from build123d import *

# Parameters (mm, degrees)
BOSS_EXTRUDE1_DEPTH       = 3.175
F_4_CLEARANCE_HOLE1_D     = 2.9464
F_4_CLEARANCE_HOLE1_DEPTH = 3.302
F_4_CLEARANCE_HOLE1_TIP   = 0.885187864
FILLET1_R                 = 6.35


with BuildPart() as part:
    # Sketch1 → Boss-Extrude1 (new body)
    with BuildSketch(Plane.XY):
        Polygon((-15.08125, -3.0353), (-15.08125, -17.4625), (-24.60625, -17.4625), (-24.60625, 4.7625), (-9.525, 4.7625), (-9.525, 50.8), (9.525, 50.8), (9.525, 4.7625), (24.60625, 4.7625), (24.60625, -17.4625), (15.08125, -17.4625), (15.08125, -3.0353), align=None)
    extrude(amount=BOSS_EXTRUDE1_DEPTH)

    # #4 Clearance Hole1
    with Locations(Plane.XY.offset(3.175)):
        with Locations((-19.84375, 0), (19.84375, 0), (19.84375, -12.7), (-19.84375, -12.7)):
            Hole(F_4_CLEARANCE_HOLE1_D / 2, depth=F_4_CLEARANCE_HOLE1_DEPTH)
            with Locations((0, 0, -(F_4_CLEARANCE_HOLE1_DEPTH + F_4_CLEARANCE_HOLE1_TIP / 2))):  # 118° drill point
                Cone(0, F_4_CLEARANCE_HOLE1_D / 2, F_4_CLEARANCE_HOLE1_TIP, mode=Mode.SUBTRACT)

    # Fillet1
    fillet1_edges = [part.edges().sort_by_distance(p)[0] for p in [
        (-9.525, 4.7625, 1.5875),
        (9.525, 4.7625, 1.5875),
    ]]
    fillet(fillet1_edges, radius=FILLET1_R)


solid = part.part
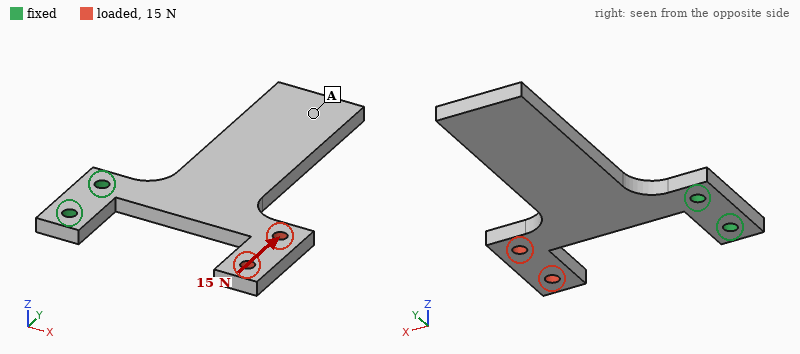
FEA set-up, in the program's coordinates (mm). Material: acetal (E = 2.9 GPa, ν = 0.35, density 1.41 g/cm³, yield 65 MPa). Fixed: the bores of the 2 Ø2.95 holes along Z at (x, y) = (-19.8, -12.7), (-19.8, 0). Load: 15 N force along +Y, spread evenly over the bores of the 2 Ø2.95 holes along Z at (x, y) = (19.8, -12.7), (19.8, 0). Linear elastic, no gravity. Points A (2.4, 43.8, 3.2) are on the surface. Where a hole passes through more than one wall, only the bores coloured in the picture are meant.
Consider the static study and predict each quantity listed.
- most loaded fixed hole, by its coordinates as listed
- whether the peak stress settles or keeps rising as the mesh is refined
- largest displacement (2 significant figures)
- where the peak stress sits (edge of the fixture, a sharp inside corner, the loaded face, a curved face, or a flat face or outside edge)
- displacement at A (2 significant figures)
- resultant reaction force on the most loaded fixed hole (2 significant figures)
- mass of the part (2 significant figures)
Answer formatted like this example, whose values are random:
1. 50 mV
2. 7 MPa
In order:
1. (-19.8, -12.7)
2. keeps rising
3. 0.83 mm
4. a sharp inside corner
5. 0.69 mm
6. 37 N
7. 6.8 g
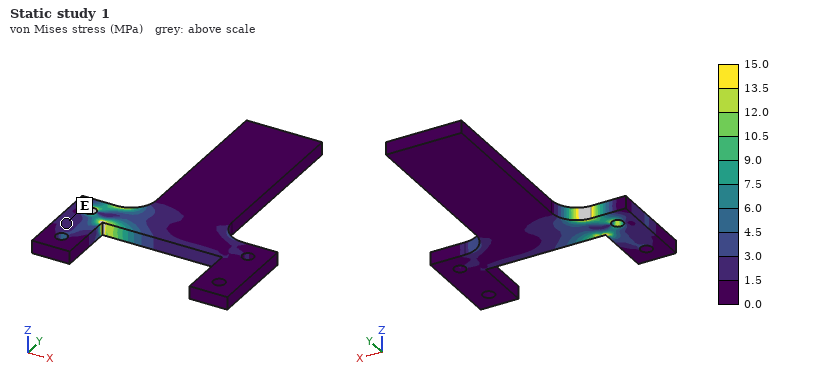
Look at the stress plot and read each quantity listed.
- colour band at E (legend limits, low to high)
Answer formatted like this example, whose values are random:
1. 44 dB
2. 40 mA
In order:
1. 1.5 to 3.0 MPa
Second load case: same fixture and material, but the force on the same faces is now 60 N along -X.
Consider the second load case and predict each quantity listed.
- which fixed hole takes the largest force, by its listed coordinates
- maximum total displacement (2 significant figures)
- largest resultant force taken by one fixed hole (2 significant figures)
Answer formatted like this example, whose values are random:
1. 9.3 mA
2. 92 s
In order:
1. (-19.8, 0)
2. 0.88 mm
3. 41 N
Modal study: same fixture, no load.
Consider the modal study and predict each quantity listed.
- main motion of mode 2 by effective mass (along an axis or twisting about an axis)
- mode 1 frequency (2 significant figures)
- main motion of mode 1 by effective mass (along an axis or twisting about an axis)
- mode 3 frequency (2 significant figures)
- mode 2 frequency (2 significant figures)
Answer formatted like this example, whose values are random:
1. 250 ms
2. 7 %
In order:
1. along Z
2. 170 Hz
3. along Z
4. 380 Hz
5. 280 Hz
